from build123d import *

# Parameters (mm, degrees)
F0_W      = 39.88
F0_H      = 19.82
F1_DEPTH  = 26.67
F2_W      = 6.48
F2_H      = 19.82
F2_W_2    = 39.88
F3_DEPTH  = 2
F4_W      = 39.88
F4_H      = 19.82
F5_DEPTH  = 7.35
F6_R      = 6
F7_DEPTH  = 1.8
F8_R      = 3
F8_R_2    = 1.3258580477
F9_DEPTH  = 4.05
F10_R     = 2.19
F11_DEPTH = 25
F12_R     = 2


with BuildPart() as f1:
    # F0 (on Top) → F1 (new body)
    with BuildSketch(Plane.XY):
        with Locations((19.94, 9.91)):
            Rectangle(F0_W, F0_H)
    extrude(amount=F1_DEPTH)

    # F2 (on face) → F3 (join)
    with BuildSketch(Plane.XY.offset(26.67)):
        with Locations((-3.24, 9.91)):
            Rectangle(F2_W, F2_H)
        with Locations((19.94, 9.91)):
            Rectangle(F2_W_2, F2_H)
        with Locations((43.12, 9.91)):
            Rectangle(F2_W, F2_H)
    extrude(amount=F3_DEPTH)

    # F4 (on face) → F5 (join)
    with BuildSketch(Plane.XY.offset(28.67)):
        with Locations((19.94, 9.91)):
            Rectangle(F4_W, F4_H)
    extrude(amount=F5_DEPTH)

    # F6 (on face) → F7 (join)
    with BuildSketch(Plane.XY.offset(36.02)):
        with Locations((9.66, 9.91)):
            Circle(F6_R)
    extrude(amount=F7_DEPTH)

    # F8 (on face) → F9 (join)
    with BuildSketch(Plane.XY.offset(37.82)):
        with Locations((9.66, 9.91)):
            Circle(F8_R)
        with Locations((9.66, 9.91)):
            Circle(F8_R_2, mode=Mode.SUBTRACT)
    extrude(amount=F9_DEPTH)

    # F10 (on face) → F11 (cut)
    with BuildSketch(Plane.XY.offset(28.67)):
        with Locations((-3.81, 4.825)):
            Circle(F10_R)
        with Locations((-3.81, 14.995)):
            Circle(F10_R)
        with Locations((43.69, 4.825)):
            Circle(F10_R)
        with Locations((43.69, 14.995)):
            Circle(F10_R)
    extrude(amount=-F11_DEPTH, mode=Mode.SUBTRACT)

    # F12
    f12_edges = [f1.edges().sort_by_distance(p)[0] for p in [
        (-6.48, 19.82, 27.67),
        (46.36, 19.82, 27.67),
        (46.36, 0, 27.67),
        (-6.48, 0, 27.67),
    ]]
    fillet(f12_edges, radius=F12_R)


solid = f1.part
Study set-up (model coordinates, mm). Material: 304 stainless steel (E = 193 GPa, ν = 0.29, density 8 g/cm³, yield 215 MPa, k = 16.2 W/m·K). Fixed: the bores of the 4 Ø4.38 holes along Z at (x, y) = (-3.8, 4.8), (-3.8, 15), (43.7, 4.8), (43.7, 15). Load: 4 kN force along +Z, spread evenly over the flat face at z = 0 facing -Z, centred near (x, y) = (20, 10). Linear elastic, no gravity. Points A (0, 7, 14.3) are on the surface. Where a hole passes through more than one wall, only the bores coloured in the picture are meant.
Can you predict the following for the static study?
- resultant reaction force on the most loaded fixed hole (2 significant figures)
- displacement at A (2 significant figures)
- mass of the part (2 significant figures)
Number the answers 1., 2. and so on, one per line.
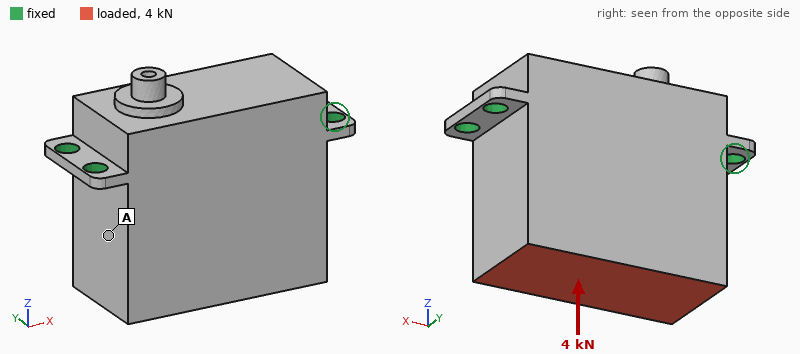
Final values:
1. 1.0 kN
2. 5.0 µm
3. 230 g
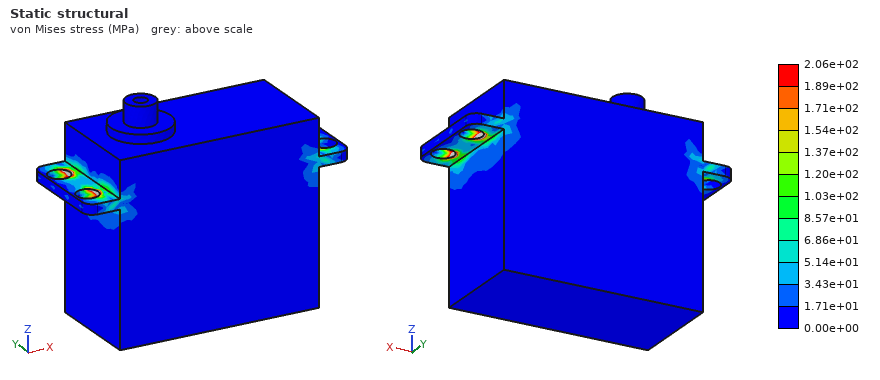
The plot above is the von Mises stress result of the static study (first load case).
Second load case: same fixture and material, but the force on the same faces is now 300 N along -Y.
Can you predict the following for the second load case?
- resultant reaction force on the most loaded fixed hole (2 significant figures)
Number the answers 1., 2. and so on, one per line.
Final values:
1. 350 N
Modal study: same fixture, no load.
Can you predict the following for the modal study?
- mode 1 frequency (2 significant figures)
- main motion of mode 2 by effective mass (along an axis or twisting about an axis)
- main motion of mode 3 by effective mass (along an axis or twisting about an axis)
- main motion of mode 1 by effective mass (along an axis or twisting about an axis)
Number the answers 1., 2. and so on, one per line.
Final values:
1. 3500 Hz
2. along Z
3. along X
4. along Y
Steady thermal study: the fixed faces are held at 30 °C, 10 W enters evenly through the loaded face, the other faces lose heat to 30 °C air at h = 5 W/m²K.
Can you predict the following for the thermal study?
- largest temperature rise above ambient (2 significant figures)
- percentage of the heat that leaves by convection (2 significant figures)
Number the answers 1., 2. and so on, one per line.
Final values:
1. 51 K
2. 9.5 %
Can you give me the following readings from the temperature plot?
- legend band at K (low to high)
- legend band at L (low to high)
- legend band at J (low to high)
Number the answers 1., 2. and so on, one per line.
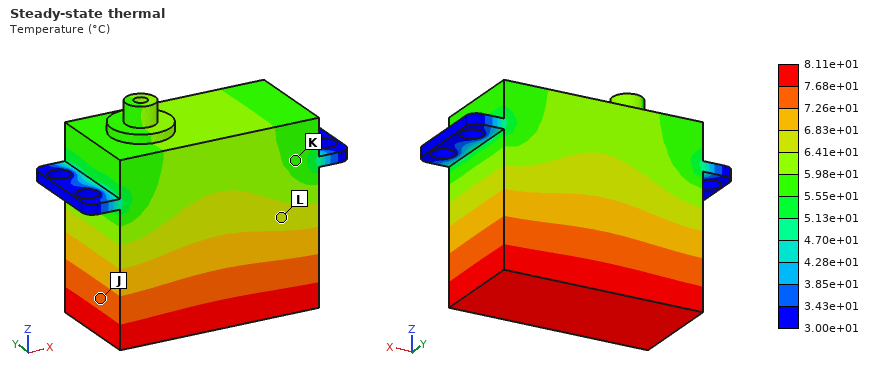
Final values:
1. 5.55e+01 to 5.98e+01 °C
2. 6.41e+01 to 6.83e+01 °C
3. 7.26e+01 to 7.68e+01 °C
